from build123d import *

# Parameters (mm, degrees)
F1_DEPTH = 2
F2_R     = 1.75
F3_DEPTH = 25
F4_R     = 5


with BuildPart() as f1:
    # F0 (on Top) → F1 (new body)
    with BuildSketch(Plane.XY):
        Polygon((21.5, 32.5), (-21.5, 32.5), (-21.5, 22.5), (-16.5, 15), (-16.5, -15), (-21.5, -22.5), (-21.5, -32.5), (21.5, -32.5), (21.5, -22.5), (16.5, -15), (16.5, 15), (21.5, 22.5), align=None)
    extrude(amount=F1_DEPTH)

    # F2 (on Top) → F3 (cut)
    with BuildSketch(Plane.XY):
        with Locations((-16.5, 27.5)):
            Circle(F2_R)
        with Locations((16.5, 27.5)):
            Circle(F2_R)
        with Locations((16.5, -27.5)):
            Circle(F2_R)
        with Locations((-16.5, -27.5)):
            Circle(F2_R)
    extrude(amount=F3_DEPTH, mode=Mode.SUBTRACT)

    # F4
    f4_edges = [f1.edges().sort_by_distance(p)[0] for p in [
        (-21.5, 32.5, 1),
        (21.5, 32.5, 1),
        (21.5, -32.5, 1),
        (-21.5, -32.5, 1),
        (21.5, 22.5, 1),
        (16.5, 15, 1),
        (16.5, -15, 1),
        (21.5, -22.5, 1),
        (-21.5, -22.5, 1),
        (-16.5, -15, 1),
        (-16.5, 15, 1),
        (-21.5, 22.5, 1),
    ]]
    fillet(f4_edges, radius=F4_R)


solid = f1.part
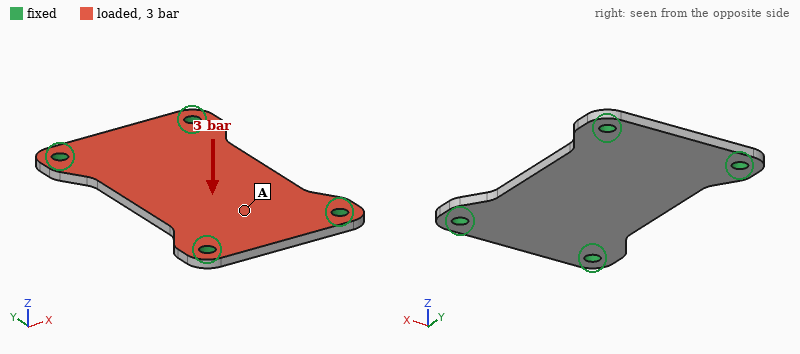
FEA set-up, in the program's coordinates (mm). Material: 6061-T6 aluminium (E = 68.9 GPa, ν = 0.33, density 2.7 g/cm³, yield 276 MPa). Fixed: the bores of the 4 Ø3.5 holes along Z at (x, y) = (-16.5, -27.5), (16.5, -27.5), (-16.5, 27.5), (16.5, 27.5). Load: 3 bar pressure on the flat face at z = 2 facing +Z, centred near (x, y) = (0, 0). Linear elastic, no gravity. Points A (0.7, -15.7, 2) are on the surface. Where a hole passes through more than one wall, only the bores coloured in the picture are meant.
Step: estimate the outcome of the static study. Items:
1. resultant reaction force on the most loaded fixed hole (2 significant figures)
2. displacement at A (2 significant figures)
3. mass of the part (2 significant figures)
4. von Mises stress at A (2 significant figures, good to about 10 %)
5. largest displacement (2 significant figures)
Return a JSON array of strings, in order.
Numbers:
["180 N", "0.10 mm", "13 g", "25 MPa", "0.18 mm"]
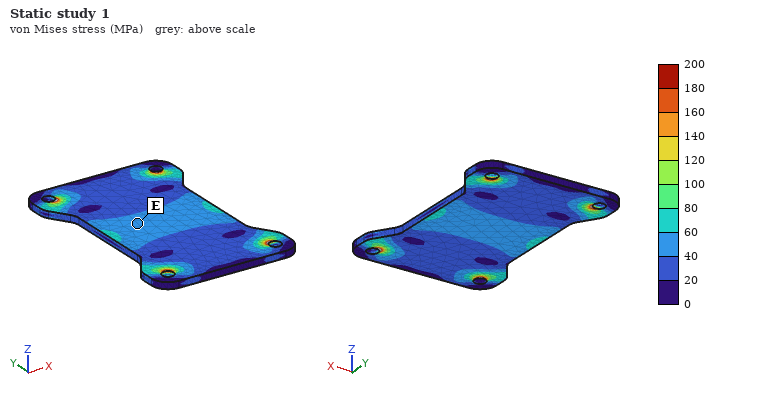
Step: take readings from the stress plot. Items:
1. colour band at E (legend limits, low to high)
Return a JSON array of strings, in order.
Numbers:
["40 to 60 MPa"]
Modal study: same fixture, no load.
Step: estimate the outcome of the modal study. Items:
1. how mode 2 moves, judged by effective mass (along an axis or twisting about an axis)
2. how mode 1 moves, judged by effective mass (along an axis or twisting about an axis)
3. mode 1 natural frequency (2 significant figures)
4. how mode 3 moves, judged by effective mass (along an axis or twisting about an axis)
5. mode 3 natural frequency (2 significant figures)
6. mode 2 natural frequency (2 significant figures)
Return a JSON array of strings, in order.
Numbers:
["twisting about Y", "along Z", "3300 Hz", "twisting about X", "8000 Hz", "5700 Hz"]
